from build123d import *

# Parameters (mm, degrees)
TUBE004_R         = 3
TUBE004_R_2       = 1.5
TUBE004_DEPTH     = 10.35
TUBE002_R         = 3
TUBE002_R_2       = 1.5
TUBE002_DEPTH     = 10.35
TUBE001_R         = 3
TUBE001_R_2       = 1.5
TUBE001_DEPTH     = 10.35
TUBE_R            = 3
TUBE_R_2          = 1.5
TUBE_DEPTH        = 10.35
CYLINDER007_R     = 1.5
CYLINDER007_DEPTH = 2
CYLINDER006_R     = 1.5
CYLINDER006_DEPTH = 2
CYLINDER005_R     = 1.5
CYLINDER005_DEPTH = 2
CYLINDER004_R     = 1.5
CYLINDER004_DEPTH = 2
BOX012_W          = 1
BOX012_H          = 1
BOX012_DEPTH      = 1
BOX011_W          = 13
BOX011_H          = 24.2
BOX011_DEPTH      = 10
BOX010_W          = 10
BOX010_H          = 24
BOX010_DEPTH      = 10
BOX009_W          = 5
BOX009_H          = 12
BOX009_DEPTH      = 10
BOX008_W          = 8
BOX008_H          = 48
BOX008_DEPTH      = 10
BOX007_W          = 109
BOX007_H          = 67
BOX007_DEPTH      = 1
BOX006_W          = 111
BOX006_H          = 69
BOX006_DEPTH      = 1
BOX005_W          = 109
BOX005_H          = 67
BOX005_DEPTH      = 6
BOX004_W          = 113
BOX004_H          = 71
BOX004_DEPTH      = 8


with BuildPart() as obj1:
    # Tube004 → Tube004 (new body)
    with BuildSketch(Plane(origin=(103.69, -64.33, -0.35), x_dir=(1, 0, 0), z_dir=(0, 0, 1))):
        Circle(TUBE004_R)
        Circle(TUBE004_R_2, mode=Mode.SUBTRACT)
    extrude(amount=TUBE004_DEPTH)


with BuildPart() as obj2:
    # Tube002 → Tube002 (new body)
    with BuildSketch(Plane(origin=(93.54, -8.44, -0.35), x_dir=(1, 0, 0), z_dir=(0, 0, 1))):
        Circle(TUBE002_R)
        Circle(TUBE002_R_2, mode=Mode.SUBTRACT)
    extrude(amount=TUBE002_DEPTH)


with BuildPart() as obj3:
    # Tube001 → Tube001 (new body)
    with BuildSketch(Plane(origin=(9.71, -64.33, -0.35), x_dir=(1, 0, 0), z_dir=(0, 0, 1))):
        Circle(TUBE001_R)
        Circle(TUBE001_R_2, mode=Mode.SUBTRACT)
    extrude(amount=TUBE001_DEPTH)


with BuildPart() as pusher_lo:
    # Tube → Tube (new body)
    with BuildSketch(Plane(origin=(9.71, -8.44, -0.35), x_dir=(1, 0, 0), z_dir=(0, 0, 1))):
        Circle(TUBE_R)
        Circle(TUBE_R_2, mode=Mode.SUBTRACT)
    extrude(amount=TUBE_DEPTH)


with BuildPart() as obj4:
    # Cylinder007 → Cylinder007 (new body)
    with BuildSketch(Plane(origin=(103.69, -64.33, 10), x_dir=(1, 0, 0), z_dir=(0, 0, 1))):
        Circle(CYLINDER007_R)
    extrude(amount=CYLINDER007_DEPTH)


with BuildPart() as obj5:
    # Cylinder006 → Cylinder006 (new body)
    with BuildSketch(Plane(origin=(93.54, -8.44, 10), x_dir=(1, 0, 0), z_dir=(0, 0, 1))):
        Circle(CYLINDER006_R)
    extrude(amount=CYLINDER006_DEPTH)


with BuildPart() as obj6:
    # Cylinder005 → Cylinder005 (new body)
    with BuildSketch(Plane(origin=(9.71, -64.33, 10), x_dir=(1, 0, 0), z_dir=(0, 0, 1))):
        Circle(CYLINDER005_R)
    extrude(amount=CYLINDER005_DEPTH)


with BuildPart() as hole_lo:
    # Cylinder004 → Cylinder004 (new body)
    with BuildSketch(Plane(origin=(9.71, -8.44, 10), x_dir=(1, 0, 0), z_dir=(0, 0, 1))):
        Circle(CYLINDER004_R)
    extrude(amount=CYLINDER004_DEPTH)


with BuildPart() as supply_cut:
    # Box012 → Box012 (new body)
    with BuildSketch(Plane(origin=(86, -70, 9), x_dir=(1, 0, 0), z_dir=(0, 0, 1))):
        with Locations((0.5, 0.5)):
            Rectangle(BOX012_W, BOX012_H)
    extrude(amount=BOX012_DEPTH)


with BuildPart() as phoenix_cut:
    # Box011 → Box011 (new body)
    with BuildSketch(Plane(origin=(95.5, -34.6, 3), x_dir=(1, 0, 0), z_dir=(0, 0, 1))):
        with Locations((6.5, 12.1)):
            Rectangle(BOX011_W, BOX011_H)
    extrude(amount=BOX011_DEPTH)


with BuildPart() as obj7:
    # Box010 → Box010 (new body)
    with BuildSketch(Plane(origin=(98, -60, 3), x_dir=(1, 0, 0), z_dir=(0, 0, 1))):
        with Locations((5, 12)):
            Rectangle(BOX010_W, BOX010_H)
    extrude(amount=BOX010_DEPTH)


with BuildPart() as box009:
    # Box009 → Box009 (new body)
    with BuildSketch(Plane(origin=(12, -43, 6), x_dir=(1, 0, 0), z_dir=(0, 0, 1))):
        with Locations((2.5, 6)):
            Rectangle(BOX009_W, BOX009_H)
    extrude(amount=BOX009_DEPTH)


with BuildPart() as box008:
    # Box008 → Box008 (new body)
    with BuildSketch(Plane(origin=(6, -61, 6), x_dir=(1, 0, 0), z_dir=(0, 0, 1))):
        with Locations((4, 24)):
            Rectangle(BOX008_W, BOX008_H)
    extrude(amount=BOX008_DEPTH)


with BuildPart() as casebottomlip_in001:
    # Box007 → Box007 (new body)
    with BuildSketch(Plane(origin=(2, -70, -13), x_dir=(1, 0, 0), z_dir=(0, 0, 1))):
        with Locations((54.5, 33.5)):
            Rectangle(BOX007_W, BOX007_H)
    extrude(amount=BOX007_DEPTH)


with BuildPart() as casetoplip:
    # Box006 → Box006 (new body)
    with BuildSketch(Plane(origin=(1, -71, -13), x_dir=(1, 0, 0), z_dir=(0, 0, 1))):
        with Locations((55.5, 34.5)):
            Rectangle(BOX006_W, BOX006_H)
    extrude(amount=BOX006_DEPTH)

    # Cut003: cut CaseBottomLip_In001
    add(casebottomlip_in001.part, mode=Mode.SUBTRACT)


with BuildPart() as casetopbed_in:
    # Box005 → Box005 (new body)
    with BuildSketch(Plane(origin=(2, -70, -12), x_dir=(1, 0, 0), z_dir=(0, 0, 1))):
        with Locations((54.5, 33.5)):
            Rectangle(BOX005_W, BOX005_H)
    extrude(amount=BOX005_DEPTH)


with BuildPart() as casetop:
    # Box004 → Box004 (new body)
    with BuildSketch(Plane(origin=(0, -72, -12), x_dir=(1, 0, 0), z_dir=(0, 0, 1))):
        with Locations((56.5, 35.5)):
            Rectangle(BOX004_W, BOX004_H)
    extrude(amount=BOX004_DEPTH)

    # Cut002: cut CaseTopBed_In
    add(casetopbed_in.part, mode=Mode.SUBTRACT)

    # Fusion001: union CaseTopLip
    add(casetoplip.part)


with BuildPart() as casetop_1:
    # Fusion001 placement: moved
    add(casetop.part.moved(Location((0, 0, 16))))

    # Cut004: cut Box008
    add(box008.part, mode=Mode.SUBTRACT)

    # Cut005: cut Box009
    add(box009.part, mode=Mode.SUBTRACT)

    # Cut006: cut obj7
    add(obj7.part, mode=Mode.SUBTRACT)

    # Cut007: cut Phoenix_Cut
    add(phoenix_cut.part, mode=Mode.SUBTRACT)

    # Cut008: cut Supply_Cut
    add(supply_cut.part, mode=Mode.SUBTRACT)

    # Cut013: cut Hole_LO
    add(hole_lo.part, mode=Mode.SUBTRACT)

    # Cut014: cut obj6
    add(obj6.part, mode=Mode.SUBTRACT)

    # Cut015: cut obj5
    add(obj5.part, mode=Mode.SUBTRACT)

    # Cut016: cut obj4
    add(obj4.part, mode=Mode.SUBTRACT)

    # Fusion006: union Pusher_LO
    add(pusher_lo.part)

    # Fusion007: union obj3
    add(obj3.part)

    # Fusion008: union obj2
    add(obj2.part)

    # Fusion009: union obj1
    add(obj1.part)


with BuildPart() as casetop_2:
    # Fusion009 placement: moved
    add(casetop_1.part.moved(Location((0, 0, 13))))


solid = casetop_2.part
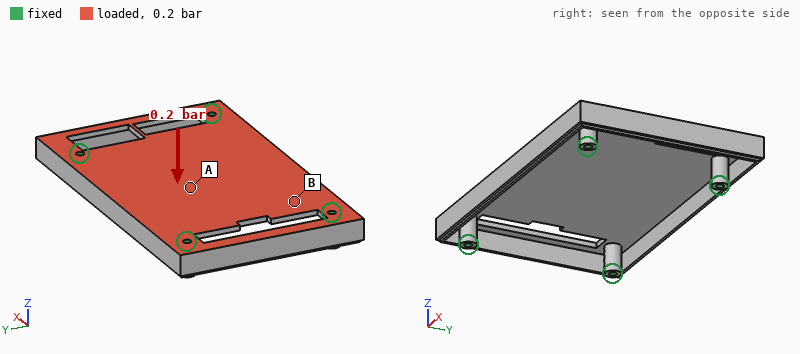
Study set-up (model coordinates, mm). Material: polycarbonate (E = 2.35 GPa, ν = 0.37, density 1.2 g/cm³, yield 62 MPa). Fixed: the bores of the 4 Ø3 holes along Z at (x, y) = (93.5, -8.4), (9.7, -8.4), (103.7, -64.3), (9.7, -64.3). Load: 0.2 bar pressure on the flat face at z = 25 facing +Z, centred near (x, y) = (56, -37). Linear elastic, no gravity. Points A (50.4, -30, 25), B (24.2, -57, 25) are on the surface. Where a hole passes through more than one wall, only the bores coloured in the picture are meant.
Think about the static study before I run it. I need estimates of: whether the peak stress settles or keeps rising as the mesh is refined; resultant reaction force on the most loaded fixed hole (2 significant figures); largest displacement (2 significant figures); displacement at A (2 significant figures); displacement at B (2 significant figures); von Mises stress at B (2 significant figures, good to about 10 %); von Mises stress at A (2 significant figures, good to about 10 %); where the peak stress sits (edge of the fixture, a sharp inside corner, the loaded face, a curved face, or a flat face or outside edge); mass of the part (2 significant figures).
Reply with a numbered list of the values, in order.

1. keeps rising
2. 42 N
3. 1.6 mm
4. 1.5 mm
5. 0.60 mm
6. 2.3 MPa
7. 7.8 MPa
8. edge of the fixture
9. 24 g
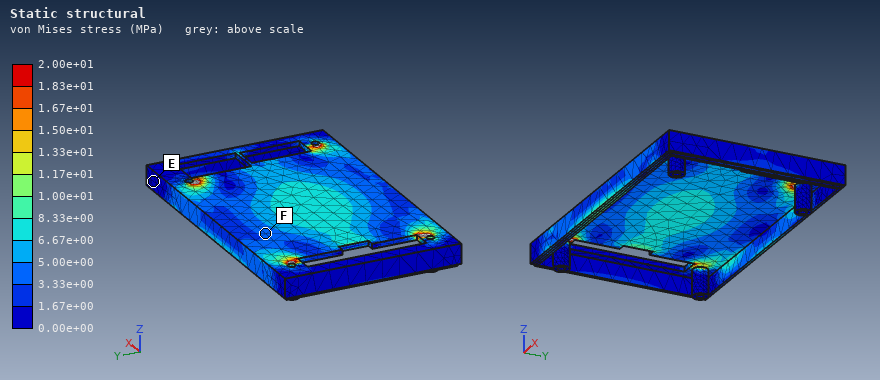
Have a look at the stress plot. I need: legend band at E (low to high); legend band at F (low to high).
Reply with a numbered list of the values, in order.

1. 0.00e+00 to 1.67e+00 MPa
2. 3.33e+00 to 5.00e+00 MPa
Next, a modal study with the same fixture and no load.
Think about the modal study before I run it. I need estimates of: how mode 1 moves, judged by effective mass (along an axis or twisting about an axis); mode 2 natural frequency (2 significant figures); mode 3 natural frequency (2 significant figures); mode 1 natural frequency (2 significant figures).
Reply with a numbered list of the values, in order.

1. along Z
2. 780 Hz
3. 860 Hz
4. 440 Hz
